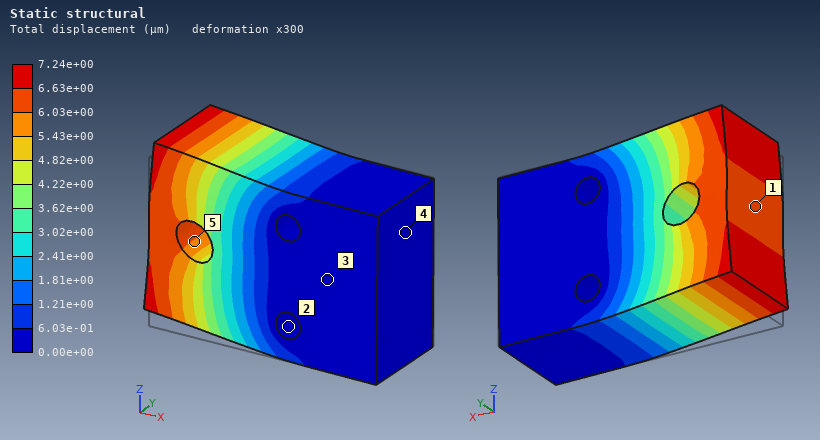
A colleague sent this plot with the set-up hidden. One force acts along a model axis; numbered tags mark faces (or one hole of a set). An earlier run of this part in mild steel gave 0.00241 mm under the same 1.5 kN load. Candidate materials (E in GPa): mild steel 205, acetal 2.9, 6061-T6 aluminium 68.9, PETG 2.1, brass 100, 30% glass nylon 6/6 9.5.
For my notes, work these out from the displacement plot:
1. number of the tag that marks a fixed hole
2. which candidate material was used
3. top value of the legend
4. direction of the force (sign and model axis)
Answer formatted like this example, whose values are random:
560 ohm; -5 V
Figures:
2; 6061-T6 aluminium; 7.24e+00 µm; +Z
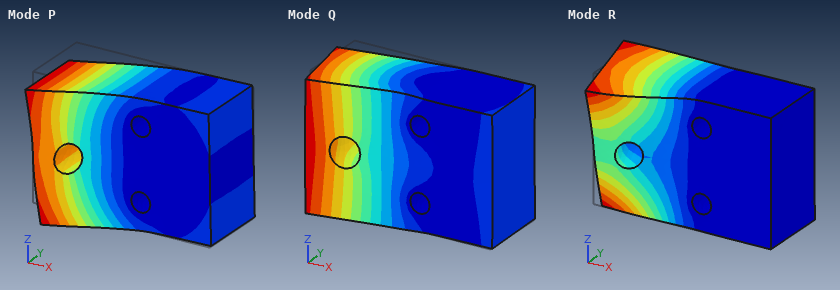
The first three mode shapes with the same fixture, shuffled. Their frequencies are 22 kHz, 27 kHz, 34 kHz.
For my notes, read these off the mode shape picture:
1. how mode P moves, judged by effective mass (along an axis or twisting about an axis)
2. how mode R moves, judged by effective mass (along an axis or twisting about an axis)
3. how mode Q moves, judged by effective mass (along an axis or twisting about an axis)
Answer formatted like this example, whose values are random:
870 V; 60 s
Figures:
along Z; twisting about X; along Y
